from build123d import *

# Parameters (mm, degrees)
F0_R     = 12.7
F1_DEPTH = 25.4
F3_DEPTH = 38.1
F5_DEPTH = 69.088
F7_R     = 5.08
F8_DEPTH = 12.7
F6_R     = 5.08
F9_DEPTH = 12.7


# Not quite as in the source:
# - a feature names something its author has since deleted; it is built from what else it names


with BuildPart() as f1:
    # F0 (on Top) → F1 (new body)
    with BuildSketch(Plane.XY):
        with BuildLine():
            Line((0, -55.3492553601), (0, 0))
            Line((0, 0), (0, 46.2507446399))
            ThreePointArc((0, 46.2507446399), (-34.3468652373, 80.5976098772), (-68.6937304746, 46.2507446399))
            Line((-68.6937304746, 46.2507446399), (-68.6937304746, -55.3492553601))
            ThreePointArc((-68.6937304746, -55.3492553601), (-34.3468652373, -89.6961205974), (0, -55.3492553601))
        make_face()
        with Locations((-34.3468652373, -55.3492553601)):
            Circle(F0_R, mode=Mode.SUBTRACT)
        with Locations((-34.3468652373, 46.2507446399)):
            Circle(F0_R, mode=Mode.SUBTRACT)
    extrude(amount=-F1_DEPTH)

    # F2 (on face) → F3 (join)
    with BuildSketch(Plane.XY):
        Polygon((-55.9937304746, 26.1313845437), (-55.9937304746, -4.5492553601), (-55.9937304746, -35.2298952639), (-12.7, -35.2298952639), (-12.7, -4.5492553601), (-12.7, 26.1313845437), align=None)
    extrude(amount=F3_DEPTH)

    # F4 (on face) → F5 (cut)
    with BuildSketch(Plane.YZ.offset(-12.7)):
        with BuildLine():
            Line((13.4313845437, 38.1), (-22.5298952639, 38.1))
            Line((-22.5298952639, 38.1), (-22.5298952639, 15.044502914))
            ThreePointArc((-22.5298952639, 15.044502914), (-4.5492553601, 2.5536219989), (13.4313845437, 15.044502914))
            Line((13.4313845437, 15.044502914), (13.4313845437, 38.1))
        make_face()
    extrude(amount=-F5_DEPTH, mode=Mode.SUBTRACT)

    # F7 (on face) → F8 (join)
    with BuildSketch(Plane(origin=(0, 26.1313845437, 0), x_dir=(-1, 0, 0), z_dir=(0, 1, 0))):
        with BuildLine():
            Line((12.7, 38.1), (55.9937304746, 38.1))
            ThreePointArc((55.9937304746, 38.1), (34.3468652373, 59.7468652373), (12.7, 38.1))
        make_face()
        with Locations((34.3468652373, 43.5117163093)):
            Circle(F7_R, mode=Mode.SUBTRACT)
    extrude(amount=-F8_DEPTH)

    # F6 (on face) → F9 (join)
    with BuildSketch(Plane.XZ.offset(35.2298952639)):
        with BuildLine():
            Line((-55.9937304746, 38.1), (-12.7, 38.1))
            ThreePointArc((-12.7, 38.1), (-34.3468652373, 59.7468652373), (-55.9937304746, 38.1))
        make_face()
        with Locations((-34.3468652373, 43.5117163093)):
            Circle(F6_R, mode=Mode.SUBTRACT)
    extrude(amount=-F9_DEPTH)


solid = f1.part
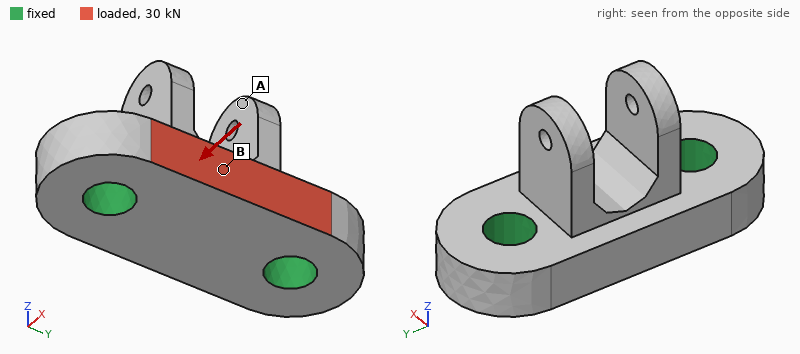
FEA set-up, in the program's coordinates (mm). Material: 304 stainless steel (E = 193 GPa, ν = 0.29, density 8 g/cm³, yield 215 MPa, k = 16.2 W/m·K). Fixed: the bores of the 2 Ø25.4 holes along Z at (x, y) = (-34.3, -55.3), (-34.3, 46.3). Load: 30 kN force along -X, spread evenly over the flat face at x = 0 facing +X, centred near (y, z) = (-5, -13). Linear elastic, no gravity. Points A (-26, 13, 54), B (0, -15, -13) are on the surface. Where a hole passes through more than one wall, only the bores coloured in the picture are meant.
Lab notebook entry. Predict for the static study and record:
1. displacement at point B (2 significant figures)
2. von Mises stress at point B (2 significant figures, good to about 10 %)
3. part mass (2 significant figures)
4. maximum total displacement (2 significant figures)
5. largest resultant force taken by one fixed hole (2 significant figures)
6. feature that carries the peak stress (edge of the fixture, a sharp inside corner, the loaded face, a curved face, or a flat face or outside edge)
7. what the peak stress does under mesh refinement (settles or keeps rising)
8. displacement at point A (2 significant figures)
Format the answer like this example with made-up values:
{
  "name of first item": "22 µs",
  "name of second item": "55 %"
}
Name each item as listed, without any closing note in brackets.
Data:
{
  "displacement at point B": "4.2 µm",
  "von Mises stress at point B": "12 MPa",
  "part mass": "2.5 kg",
  "maximum total displacement": "4.8 µm",
  "largest resultant force taken by one fixed hole": "15 kN",
  "feature that carries the peak stress": "edge of the fixture",
  "what the peak stress does under mesh refinement": "keeps rising",
  "displacement at point A": "2.9 µm"
}
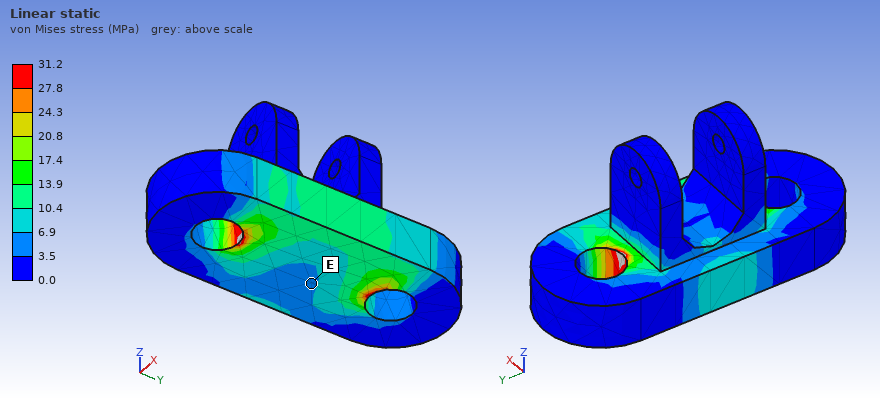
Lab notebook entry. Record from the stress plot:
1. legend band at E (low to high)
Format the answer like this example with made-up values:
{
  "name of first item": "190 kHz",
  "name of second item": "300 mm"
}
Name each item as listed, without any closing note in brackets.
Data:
{
  "legend band at E": "3.5 to 6.9 MPa"
}
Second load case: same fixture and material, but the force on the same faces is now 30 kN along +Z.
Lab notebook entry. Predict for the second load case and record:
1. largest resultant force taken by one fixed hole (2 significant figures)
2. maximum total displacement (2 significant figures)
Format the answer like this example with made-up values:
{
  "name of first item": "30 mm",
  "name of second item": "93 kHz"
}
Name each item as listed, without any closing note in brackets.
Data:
{
  "largest resultant force taken by one fixed hole": "15 kN",
  "maximum total displacement": "25 µm"
}
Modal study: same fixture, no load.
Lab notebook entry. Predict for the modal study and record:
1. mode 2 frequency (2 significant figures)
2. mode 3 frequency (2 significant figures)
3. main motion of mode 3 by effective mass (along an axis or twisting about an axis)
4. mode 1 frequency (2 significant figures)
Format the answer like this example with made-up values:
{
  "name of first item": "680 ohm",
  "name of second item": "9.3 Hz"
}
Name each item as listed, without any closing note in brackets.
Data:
{
  "mode 2 frequency": "3900 Hz",
  "mode 3 frequency": "5500 Hz",
  "main motion of mode 3 by effective mass": "along X",
  "mode 1 frequency": "3800 Hz"
}
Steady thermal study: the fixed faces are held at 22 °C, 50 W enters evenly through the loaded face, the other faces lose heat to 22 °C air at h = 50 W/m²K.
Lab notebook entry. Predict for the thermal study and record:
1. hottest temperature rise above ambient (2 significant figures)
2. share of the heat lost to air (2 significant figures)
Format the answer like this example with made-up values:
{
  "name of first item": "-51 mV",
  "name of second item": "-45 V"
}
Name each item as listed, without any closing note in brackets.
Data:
{
  "hottest temperature rise above ambient": "38 K",
  "share of the heat lost to air": "25 %"
}
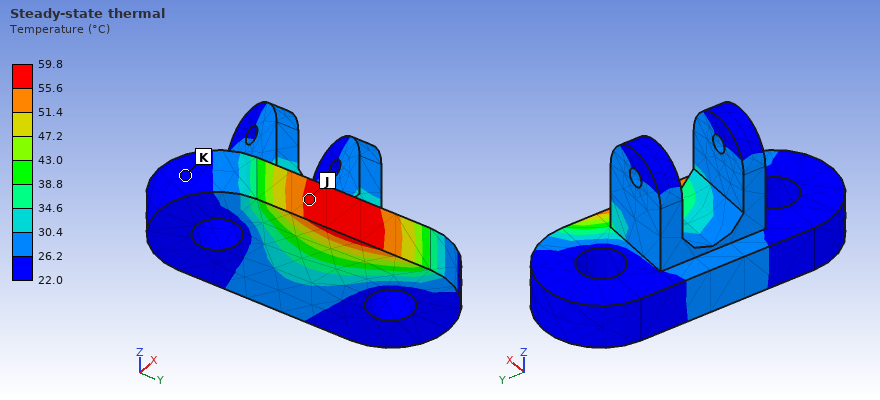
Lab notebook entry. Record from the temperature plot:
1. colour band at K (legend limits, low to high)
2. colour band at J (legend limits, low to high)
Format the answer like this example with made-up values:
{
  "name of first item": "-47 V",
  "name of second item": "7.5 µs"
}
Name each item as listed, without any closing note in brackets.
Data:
{
  "colour band at K": "22.0 to 26.2 °C",
  "colour band at J": "55.6 to 59.8 °C"
}
